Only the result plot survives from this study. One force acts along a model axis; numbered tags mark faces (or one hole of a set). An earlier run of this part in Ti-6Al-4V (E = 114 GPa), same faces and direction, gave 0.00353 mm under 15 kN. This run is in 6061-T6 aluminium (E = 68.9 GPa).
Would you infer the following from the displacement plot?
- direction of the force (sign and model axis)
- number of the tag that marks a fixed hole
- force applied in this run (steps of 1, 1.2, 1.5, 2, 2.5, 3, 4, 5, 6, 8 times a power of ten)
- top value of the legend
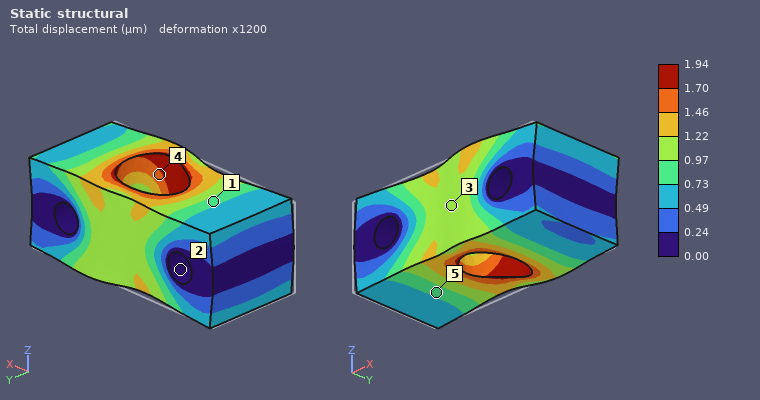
+X
2
5 kN
1.94 µm
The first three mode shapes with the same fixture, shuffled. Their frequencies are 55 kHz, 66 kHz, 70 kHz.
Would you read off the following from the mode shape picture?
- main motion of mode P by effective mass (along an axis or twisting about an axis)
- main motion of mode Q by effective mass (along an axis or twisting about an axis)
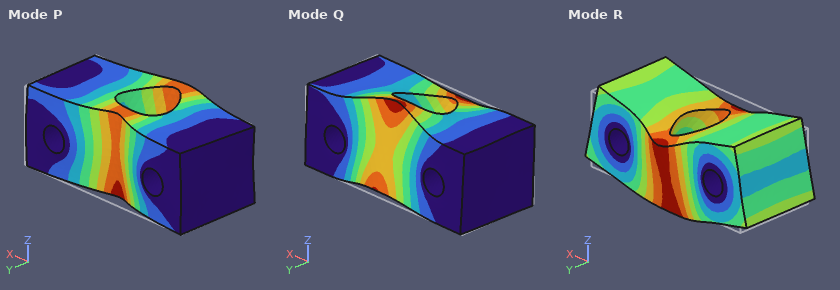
along Y
twisting about X
